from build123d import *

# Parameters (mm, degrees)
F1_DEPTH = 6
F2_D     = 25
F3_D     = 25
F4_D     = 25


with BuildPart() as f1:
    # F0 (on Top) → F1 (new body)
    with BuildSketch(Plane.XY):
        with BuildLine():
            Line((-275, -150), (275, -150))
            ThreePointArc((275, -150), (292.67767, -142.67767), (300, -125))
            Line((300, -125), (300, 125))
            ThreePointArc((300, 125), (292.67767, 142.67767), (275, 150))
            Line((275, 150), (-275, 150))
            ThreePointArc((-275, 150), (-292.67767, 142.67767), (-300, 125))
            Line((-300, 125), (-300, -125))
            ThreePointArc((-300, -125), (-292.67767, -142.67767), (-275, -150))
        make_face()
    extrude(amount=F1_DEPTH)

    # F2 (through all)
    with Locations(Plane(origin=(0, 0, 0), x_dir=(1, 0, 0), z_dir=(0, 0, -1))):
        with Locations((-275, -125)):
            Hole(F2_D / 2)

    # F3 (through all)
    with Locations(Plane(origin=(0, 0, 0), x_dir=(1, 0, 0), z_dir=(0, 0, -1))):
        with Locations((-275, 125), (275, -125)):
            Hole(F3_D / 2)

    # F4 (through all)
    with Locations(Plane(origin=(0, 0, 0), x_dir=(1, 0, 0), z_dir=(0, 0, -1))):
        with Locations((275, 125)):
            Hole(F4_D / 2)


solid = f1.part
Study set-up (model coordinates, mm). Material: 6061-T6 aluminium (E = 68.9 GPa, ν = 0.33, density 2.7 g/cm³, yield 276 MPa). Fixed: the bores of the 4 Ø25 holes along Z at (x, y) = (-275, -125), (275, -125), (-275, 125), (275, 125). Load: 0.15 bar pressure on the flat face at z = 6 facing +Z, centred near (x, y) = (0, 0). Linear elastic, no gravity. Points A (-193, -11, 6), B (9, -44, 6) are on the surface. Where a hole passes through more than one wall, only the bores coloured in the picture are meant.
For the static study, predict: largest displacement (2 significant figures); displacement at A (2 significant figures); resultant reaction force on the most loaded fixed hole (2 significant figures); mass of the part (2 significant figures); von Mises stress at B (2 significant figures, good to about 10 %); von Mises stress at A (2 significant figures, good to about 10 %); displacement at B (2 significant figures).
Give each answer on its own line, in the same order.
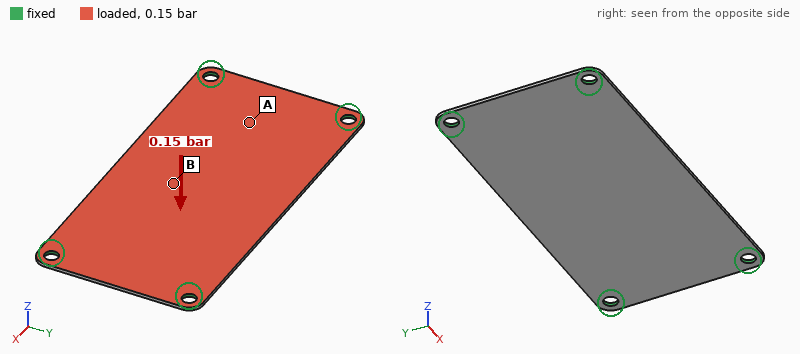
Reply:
3.3 mm
1.1 mm
670 N
2.9 kg
30 MPa
13 MPa
3.1 mm
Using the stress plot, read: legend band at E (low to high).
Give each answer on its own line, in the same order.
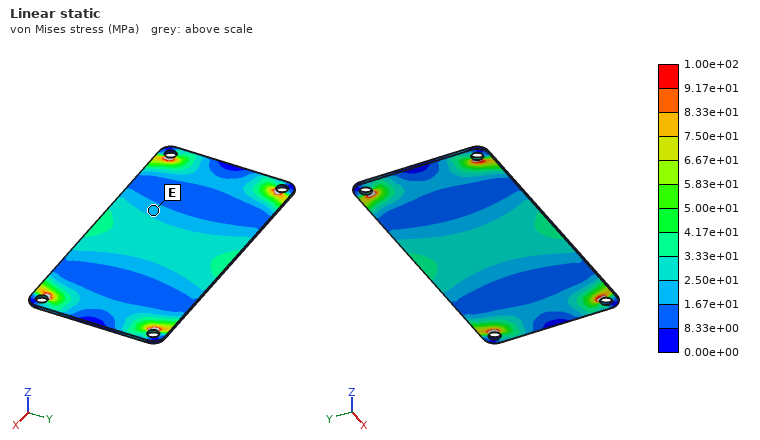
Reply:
1.67e+01 to 2.50e+01 MPa
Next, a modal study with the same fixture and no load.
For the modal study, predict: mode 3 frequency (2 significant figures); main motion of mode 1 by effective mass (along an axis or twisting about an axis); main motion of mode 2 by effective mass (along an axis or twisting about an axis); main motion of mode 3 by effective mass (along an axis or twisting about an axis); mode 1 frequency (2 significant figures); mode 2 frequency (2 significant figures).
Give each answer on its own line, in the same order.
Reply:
270 Hz
along Z
twisting about X
twisting about Y
98 Hz
170 Hz
